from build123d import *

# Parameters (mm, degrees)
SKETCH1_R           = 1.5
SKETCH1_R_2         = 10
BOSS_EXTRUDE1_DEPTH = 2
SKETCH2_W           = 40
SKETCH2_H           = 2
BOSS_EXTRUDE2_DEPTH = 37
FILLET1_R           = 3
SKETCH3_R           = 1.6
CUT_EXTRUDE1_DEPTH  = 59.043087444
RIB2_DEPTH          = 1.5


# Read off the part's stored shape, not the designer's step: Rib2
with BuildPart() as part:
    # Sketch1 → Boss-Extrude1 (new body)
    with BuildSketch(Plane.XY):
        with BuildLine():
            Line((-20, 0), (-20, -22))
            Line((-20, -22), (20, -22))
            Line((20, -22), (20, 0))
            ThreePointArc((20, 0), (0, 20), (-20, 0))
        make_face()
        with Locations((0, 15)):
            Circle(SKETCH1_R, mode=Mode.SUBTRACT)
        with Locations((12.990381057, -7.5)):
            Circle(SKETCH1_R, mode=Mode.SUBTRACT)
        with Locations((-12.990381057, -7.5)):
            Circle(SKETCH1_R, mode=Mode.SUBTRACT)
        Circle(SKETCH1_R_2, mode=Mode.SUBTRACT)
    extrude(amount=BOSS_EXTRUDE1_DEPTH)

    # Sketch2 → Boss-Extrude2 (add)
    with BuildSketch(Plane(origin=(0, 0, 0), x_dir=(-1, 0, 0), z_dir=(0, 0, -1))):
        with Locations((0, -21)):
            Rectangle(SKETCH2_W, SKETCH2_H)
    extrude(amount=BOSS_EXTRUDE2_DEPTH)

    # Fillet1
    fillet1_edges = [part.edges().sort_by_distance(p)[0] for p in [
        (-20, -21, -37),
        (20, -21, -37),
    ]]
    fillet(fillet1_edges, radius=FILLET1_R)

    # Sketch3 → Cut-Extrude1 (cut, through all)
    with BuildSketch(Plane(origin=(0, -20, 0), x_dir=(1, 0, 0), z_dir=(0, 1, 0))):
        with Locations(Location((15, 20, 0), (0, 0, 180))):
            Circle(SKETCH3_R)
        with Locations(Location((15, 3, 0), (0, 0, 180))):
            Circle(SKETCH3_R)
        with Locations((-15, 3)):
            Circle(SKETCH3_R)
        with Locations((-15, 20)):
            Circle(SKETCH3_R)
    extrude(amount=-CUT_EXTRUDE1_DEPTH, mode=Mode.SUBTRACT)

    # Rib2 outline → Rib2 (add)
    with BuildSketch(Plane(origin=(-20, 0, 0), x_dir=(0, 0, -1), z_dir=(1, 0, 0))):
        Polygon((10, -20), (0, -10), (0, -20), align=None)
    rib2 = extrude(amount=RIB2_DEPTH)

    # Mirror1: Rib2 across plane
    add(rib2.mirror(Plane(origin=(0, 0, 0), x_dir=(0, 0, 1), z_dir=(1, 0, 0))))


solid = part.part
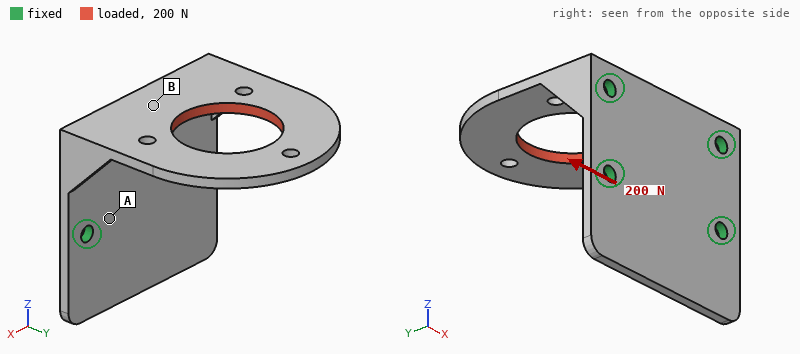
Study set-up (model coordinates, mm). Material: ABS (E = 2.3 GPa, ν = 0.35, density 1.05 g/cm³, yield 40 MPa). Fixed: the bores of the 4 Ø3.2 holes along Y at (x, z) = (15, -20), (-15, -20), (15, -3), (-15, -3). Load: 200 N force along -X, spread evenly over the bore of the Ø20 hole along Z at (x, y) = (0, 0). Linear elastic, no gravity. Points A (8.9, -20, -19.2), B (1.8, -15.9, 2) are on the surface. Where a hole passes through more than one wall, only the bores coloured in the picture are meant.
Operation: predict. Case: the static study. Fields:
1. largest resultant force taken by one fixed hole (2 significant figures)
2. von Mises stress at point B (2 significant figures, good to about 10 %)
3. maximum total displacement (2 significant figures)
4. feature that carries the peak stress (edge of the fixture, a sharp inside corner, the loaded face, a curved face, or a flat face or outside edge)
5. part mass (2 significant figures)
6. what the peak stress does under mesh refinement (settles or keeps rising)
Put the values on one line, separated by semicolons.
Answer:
170 N; 5.9 MPa; 0.61 mm; edge of the fixture; 5.7 g; keeps rising
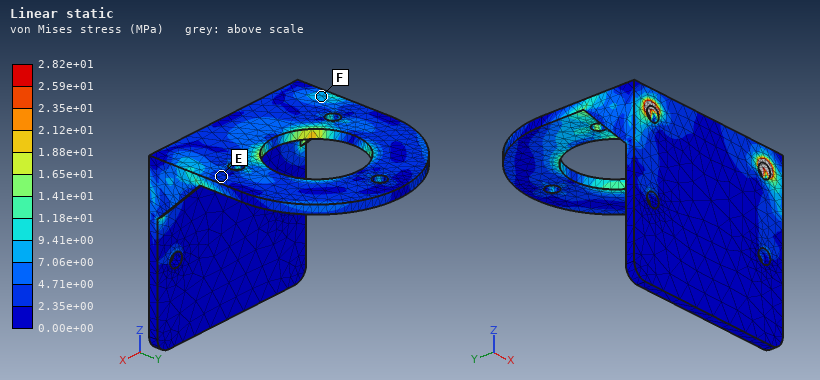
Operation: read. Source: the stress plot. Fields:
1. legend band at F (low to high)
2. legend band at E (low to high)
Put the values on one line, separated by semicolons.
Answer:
7.06e+00 to 9.41e+00 MPa; 2.35e+00 to 4.71e+00 MPa
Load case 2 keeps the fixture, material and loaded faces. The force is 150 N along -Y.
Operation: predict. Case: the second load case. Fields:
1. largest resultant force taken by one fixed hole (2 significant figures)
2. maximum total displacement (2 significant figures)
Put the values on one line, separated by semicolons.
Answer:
81 N; 0.49 mm
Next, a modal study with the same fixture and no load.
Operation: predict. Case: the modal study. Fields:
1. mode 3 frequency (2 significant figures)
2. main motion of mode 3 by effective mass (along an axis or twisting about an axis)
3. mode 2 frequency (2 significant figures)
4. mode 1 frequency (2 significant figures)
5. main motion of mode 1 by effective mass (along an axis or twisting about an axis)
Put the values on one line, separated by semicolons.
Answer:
1500 Hz; along Y; 1000 Hz; 370 Hz; along Z
